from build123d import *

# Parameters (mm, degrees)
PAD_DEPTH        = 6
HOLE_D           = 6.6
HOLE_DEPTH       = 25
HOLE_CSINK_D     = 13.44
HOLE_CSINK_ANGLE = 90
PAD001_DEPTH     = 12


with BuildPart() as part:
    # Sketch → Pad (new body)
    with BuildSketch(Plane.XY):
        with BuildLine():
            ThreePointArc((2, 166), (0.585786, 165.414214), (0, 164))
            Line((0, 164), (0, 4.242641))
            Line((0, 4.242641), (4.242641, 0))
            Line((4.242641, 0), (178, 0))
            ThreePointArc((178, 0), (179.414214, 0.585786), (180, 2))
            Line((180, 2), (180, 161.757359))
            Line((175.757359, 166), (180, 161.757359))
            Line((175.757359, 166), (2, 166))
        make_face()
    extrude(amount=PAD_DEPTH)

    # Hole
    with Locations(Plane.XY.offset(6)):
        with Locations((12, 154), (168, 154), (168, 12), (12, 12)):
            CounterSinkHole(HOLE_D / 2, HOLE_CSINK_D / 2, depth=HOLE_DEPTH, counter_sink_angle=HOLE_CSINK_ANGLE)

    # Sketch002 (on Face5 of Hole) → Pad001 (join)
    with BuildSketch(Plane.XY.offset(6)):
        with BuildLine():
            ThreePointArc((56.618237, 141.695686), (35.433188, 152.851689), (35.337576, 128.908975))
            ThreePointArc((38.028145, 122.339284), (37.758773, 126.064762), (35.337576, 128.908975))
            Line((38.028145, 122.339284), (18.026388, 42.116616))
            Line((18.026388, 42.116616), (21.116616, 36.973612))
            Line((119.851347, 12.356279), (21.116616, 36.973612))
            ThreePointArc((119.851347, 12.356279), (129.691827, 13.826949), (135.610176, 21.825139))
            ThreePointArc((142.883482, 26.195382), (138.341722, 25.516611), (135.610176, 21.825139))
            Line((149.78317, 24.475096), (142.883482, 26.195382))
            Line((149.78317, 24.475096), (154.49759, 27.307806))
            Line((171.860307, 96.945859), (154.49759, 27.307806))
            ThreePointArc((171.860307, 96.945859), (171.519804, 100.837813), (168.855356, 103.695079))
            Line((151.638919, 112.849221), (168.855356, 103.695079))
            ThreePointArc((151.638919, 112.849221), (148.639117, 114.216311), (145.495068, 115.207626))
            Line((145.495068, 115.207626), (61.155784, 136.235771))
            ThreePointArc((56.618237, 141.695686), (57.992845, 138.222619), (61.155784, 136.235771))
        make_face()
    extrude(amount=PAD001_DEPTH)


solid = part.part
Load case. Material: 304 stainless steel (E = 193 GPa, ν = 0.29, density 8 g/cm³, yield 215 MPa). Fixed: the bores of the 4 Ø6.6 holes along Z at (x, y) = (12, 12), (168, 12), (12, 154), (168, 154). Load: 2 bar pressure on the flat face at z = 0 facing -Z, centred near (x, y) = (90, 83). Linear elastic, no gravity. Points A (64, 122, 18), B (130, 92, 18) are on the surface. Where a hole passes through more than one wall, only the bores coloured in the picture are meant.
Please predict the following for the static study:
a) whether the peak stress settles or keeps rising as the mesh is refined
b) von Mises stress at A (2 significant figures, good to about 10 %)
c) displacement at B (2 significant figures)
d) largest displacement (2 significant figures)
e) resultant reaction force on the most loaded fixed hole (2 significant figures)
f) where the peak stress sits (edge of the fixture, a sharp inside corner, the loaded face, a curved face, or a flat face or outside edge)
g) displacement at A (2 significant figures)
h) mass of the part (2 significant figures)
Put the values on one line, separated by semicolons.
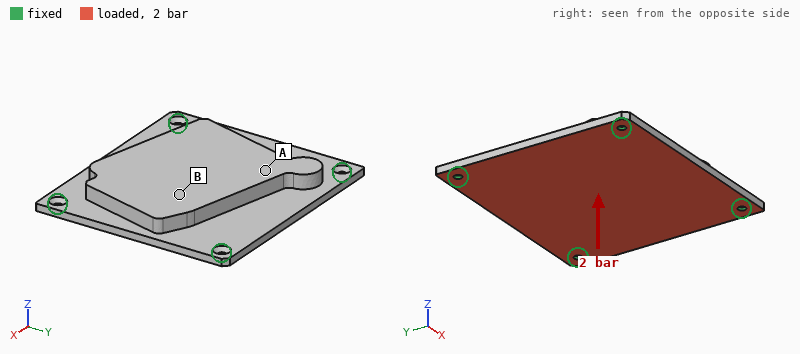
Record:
keeps rising; 21 MPa; 55 µm; 64 µm; 3.8 kN; edge of the fixture; 49 µm; 2.8 kg
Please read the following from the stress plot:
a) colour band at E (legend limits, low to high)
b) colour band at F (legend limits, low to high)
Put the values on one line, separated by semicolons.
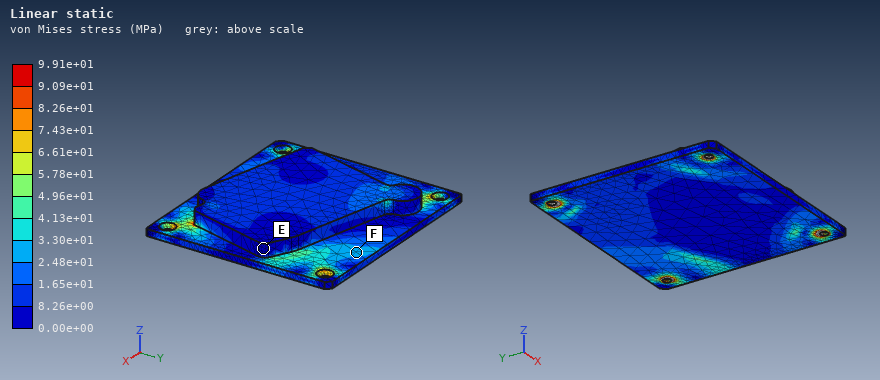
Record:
0.00e+00 to 8.26e+00 MPa; 2.48e+01 to 3.30e+01 MPa
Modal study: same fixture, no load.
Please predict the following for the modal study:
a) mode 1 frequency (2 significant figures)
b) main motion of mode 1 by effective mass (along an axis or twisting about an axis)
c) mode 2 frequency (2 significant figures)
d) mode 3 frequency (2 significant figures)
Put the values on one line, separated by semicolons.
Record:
1000 Hz; along Z; 1600 Hz; 1900 Hz
